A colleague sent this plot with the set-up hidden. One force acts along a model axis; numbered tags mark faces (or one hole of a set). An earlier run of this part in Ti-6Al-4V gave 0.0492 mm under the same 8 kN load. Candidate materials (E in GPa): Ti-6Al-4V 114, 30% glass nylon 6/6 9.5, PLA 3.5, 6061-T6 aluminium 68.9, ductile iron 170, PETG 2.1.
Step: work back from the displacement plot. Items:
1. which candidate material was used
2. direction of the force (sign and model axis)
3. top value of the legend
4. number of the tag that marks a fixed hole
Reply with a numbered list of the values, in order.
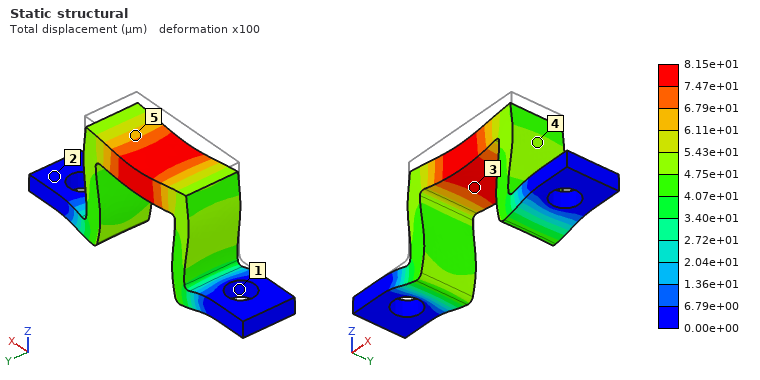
1. 6061-T6 aluminium
2. -Z
3. 8.15e+01 µm
4. 1
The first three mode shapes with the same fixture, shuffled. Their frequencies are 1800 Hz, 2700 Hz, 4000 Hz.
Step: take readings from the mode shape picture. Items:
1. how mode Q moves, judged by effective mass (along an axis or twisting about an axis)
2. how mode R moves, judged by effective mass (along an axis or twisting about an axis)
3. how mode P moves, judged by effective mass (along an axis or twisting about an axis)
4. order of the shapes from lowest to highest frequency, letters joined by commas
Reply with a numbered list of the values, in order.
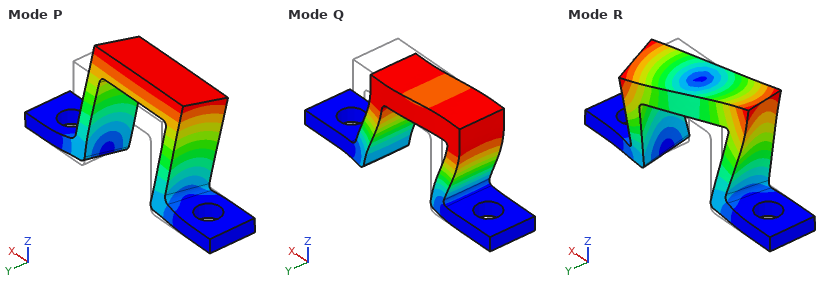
1. along X
2. twisting about Z
3. along Y
4. P, Q, R
